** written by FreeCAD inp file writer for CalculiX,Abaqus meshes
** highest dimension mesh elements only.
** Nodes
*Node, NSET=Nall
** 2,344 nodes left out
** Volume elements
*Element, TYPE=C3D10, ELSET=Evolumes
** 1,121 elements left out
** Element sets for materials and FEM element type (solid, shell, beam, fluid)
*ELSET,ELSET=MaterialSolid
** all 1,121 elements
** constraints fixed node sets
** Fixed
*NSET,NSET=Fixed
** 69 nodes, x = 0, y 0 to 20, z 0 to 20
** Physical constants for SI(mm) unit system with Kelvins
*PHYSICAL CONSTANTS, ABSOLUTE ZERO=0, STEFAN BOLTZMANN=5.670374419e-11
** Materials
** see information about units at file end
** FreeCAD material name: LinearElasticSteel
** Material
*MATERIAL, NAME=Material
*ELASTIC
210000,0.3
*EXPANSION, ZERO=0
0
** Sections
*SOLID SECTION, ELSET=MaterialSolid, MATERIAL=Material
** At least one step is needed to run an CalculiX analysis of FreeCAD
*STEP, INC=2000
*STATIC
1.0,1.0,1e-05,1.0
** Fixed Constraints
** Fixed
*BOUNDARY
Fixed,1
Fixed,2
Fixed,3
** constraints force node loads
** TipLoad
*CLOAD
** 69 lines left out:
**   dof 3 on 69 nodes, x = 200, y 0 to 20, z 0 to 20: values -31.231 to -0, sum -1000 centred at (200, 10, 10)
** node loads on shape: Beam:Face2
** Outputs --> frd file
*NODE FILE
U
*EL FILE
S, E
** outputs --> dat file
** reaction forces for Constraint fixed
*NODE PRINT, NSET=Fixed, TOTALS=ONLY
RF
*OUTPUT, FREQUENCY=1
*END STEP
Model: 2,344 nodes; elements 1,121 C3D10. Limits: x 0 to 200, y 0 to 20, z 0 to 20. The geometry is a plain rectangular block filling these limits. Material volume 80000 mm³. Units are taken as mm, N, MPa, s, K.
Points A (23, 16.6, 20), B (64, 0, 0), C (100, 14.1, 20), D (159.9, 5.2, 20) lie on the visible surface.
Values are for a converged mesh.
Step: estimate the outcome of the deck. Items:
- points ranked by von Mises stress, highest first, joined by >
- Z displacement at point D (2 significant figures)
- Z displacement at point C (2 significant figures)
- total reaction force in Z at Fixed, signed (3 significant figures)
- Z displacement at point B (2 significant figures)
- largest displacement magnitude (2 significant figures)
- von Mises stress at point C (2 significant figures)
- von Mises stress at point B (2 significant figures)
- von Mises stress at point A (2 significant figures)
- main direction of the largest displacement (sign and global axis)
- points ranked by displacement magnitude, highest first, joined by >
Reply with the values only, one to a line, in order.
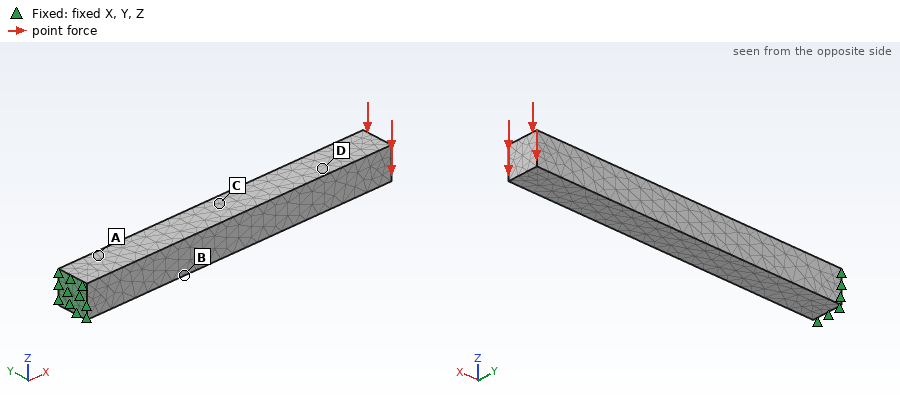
A > B > C > D
-0.67 mm
-0.30 mm
1000 N
-0.13 mm
0.96 mm
75 MPa
100 MPa
130 MPa
-Z
D > C > B > A
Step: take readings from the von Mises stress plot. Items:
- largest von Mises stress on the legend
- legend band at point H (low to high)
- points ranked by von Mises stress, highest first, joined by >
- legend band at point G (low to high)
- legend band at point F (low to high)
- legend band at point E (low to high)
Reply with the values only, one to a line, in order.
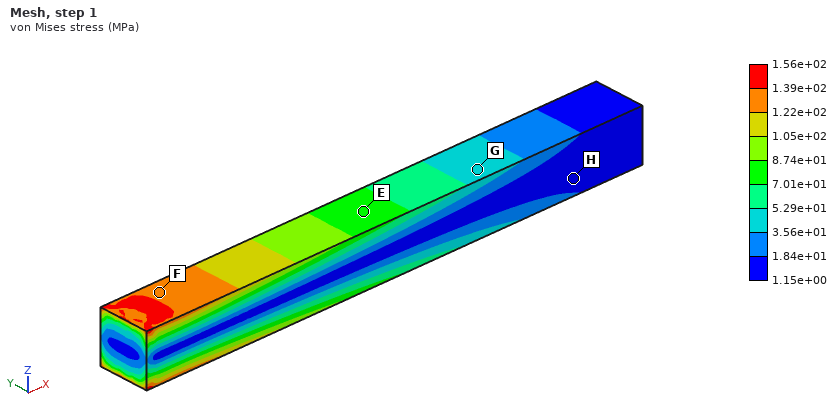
1.56e+02 MPa
1.15e+00 to 1.84e+01 MPa
F > E > G > H
3.56e+01 to 5.29e+01 MPa
1.22e+02 to 1.39e+02 MPa
7.01e+01 to 8.74e+01 MPa
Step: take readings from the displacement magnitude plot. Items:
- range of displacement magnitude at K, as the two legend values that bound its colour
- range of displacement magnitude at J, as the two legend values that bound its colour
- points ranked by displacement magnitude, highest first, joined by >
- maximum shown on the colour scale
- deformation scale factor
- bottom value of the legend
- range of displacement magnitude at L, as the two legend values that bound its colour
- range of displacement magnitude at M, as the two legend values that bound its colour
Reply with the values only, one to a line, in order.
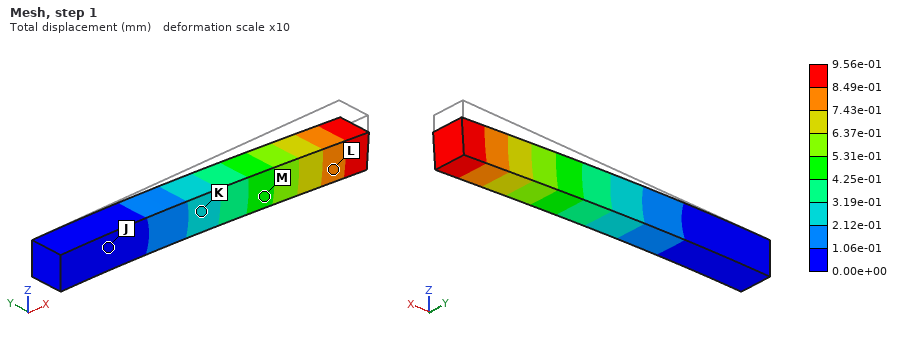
2.12e-01 to 3.19e-01 mm
0.00e+00 to 1.06e-01 mm
L > M > K > J
9.56e-01 mm
10
0.00e+00 mm
7.43e-01 to 8.49e-01 mm
4.25e-01 to 5.31e-01 mm
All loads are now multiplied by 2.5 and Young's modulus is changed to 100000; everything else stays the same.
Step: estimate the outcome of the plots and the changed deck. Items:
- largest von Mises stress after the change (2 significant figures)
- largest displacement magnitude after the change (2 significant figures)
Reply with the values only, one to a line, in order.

390 MPa
5.0 mm
